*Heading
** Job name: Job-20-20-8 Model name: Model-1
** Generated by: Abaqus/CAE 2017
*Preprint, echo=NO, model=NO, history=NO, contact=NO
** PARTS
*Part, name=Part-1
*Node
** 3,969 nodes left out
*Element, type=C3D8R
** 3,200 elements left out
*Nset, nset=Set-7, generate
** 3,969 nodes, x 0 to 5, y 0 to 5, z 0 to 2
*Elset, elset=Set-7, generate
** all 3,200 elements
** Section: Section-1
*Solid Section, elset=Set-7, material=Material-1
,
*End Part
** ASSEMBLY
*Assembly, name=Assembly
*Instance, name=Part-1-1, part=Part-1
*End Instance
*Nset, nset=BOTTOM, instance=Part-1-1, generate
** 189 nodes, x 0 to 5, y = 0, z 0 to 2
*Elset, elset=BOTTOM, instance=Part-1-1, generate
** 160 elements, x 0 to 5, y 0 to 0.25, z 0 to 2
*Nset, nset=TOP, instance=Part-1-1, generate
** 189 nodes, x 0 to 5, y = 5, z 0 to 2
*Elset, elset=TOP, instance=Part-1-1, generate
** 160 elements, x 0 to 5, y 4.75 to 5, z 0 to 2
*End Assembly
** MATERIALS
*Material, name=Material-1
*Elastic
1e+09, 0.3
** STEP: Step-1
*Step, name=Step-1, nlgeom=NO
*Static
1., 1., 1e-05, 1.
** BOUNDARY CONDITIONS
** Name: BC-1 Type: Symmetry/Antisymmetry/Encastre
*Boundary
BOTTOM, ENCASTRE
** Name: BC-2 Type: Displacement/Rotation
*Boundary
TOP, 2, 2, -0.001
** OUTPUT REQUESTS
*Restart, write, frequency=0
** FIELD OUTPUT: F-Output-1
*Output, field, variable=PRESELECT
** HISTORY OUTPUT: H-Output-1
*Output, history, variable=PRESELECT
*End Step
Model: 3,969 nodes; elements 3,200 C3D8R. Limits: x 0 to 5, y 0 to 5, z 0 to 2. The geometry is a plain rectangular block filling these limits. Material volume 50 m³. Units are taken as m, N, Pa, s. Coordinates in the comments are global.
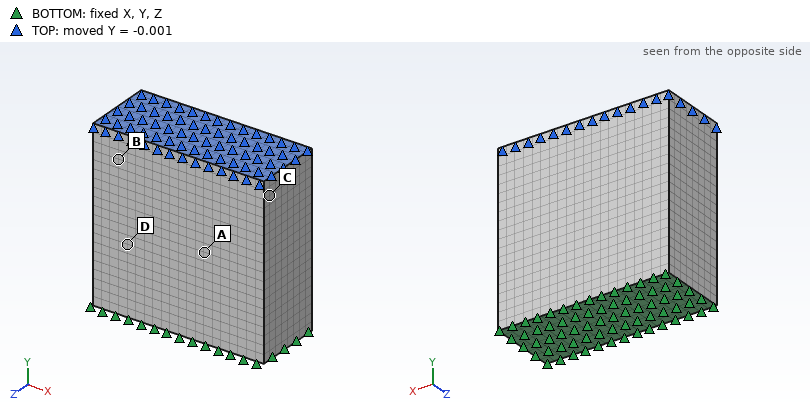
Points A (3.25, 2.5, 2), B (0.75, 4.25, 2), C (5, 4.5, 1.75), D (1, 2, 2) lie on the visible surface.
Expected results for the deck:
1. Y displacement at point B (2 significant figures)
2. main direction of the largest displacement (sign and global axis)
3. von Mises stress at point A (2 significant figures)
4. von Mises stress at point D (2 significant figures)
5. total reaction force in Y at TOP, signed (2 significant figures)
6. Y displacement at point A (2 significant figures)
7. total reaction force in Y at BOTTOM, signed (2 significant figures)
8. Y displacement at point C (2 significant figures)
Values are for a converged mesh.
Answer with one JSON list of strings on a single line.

["-8.5e-04 m", "-Y", "2.1e+05 Pa", "2.0e+05 Pa", "-2.0e+06 N", "-4.8e-04 m", "2.0e+06 N", "-9.0e-04 m"]
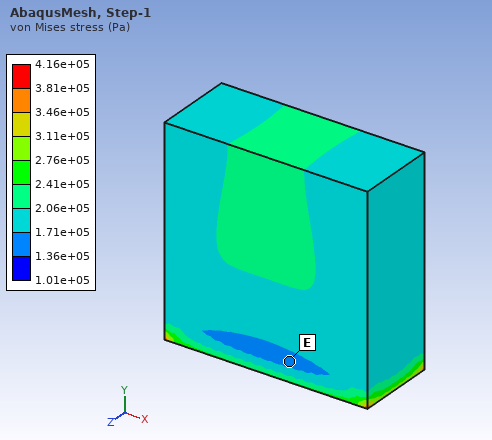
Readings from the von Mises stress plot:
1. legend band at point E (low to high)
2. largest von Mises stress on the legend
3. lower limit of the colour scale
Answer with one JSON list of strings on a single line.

["1.36e+05 to 1.71e+05 Pa", "4.16e+05 Pa", "1.01e+05 Pa"]
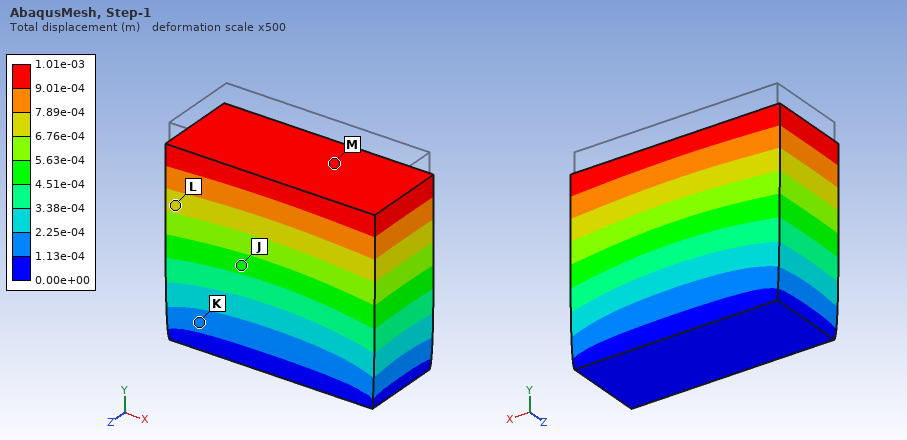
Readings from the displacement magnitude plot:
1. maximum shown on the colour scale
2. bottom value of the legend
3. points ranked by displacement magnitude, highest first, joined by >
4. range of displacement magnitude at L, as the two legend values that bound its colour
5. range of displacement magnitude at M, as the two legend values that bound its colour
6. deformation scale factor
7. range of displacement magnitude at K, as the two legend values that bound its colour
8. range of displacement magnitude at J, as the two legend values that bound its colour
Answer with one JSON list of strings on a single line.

["1.01e-03 m", "0.00e+00 m", "M > L > J > K", "6.76e-04 to 7.89e-04 m", "9.01e-04 to 1.01e-03 m", "500", "1.13e-04 to 2.25e-04 m", "4.51e-04 to 5.63e-04 m"]
